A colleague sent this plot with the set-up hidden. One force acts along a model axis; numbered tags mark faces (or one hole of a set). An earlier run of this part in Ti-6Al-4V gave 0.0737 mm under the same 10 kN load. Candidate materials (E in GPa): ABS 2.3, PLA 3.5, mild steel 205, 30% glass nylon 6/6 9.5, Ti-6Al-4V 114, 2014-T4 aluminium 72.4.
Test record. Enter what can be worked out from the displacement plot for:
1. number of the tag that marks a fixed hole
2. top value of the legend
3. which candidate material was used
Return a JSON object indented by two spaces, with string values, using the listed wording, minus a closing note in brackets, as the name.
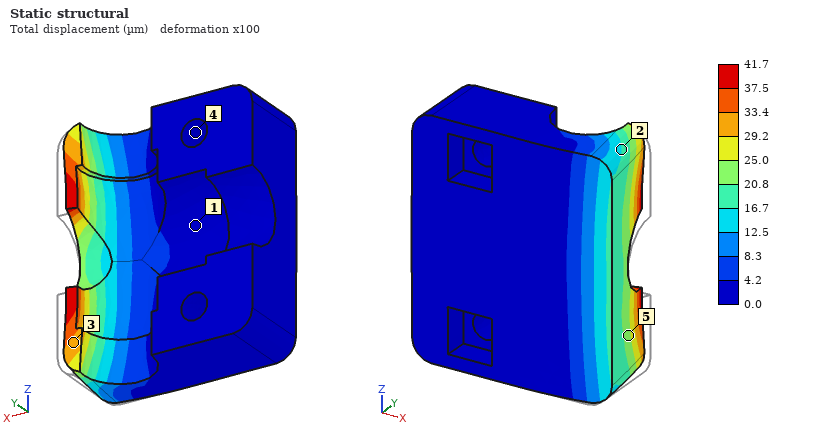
{
  "number of the tag that marks a fixed hole": "4",
  "top value of the legend": "41.7 µm",
  "which candidate material was used": "mild steel"
}
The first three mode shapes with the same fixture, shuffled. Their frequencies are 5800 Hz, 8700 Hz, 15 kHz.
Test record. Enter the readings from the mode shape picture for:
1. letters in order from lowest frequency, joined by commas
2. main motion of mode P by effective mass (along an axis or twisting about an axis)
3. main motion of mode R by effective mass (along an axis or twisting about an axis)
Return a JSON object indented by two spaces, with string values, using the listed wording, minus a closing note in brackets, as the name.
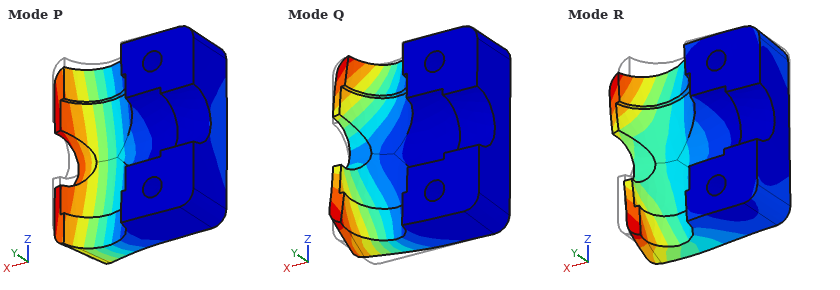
{
  "letters in order from lowest frequency, joined by commas": "P, Q, R",
  "main motion of mode P by effective mass": "along Y",
  "main motion of mode R by effective mass": "along Z"
}
